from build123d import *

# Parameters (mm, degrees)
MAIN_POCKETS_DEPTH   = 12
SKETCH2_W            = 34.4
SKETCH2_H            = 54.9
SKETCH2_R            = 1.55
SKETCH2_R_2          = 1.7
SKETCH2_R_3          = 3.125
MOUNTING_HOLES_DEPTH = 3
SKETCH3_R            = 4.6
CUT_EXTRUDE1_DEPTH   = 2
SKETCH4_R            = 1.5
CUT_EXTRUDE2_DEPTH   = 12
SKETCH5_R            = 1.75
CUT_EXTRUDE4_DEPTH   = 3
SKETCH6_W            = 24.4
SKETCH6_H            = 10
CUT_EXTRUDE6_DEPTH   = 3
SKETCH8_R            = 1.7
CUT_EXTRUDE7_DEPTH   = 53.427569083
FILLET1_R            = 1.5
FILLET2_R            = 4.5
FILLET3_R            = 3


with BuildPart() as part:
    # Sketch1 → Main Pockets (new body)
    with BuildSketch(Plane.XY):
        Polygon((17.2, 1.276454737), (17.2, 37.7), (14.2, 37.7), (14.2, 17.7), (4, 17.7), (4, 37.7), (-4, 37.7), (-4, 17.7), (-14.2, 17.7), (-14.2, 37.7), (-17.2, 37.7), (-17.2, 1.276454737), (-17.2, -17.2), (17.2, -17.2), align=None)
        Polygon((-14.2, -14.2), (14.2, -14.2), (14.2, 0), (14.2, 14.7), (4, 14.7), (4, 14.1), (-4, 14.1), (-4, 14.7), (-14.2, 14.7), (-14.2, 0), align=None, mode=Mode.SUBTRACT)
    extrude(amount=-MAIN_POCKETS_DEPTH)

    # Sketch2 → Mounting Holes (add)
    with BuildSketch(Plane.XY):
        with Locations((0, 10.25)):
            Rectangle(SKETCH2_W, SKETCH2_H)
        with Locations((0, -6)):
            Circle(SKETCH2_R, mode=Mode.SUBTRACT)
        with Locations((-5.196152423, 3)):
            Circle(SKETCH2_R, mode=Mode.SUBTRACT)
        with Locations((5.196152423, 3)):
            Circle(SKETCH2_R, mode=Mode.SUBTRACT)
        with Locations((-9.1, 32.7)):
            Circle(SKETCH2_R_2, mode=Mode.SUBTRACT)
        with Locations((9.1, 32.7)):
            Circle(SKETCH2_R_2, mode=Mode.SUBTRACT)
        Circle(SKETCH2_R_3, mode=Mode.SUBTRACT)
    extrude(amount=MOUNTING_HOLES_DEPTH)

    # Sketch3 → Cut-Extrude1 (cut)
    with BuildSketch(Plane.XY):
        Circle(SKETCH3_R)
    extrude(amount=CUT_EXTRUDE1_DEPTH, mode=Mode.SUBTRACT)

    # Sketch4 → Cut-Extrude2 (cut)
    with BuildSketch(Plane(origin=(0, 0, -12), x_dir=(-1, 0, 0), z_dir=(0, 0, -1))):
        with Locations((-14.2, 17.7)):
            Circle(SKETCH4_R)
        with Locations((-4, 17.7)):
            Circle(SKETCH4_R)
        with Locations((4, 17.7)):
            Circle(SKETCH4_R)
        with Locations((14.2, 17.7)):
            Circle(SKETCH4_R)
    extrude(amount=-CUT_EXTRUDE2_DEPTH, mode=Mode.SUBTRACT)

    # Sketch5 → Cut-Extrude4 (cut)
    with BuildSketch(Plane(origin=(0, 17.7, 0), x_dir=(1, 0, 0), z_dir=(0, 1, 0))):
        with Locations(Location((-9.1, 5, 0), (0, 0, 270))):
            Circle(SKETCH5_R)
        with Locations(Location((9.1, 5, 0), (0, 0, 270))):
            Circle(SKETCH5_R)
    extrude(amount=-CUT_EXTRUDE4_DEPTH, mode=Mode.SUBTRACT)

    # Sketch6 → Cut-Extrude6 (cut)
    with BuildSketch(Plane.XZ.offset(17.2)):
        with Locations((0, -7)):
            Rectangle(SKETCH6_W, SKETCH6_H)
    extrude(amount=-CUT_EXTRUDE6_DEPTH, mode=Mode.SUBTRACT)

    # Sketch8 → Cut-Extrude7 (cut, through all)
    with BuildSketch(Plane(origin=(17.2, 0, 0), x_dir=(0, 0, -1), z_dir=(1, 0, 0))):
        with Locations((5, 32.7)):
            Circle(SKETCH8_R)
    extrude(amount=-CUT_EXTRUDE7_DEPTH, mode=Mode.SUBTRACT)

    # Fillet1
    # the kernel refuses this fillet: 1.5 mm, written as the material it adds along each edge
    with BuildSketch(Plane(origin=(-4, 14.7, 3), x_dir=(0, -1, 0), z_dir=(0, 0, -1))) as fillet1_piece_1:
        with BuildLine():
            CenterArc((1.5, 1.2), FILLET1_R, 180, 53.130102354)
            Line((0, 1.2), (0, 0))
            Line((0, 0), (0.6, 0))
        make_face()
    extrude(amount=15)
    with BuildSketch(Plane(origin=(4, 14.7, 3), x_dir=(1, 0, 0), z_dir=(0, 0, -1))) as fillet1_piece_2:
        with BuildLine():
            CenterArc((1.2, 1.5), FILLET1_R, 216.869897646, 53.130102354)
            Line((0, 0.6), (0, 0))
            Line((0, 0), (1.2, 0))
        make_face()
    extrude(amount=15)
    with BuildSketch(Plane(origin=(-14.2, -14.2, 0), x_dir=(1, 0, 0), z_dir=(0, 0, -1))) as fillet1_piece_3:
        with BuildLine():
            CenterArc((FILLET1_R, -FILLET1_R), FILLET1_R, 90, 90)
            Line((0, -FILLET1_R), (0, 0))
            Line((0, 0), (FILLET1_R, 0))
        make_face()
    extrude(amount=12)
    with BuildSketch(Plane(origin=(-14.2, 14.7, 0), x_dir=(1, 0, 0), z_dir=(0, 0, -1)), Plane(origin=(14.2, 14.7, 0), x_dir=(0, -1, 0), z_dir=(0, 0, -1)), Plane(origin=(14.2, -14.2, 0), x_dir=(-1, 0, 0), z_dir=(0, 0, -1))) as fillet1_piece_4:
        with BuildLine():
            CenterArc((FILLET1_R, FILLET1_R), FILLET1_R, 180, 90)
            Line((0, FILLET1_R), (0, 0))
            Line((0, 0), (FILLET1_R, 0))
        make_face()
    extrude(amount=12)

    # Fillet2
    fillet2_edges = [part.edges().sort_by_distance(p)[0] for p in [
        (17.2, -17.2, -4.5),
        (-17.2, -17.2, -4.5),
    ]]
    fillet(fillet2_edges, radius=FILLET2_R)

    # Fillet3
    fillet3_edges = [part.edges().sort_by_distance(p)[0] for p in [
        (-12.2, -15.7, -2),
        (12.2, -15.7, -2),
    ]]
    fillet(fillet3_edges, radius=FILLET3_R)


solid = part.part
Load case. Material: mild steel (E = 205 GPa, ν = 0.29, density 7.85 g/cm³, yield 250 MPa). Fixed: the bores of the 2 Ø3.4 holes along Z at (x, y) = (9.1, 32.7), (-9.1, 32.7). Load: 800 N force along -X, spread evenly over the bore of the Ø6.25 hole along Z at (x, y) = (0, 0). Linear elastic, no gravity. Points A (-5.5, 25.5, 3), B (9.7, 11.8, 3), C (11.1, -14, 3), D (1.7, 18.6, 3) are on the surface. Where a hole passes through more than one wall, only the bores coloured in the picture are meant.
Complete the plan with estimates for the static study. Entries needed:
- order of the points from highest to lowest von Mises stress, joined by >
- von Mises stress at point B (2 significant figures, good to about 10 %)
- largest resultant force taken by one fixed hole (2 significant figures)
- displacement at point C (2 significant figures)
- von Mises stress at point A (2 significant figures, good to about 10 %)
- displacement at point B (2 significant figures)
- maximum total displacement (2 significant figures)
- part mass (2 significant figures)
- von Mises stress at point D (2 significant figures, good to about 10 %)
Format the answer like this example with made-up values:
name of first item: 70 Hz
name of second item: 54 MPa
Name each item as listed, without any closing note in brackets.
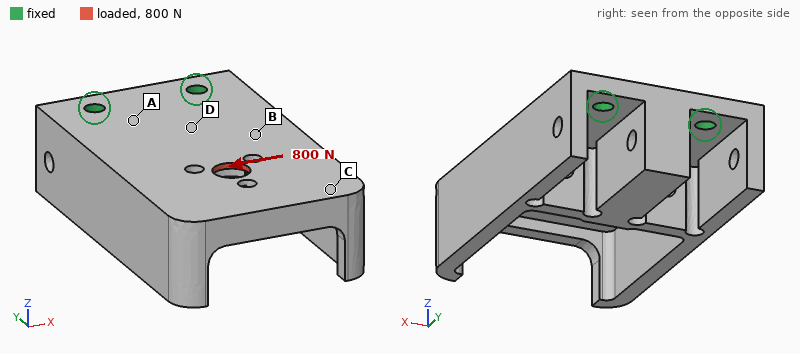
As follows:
order of the points from highest to lowest von Mises stress, joined by >: A > D > B > C
von Mises stress at point B: 16 MPa
largest resultant force taken by one fixed hole: 1.3 kN
displacement at point C: 16 µm
von Mises stress at point A: 35 MPa
displacement at point B: 7.0 µm
maximum total displacement: 17 µm
part mass: 95 g
von Mises stress at point D: 26 MPa
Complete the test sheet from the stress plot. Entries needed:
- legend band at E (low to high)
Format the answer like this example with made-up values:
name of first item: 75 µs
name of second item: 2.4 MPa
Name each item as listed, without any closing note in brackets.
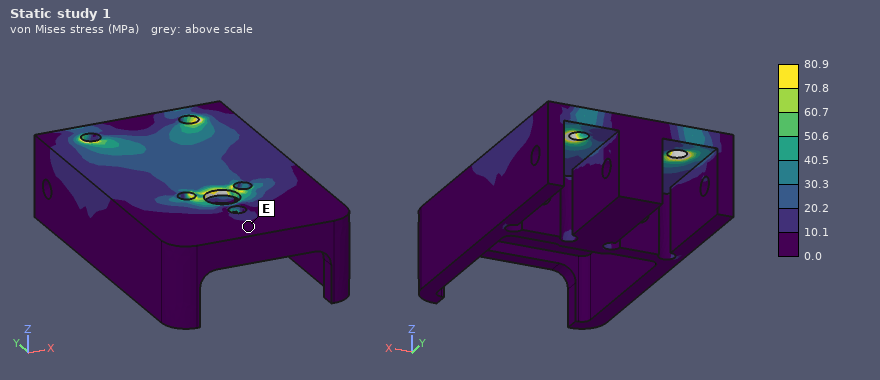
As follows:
legend band at E: 0.0 to 10.1 MPa
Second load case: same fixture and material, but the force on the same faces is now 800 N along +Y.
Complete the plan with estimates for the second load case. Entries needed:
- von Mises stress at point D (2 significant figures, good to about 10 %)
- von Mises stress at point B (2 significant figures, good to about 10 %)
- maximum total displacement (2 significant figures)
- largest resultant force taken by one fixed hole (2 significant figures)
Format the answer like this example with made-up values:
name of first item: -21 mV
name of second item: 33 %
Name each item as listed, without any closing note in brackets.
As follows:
von Mises stress at point D: 8.6 MPa
von Mises stress at point B: 10.0 MPa
maximum total displacement: 11 µm
largest resultant force taken by one fixed hole: 400 N
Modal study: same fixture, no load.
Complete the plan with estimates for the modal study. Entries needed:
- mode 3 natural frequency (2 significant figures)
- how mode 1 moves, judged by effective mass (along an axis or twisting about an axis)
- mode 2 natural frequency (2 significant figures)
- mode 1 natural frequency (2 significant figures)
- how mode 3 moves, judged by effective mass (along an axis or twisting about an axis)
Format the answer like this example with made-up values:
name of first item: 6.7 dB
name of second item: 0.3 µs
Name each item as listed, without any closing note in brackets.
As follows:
mode 3 natural frequency: 5600 Hz
how mode 1 moves, judged by effective mass: along Z
mode 2 natural frequency: 3100 Hz
mode 1 natural frequency: 1600 Hz
how mode 3 moves, judged by effective mass: along X
